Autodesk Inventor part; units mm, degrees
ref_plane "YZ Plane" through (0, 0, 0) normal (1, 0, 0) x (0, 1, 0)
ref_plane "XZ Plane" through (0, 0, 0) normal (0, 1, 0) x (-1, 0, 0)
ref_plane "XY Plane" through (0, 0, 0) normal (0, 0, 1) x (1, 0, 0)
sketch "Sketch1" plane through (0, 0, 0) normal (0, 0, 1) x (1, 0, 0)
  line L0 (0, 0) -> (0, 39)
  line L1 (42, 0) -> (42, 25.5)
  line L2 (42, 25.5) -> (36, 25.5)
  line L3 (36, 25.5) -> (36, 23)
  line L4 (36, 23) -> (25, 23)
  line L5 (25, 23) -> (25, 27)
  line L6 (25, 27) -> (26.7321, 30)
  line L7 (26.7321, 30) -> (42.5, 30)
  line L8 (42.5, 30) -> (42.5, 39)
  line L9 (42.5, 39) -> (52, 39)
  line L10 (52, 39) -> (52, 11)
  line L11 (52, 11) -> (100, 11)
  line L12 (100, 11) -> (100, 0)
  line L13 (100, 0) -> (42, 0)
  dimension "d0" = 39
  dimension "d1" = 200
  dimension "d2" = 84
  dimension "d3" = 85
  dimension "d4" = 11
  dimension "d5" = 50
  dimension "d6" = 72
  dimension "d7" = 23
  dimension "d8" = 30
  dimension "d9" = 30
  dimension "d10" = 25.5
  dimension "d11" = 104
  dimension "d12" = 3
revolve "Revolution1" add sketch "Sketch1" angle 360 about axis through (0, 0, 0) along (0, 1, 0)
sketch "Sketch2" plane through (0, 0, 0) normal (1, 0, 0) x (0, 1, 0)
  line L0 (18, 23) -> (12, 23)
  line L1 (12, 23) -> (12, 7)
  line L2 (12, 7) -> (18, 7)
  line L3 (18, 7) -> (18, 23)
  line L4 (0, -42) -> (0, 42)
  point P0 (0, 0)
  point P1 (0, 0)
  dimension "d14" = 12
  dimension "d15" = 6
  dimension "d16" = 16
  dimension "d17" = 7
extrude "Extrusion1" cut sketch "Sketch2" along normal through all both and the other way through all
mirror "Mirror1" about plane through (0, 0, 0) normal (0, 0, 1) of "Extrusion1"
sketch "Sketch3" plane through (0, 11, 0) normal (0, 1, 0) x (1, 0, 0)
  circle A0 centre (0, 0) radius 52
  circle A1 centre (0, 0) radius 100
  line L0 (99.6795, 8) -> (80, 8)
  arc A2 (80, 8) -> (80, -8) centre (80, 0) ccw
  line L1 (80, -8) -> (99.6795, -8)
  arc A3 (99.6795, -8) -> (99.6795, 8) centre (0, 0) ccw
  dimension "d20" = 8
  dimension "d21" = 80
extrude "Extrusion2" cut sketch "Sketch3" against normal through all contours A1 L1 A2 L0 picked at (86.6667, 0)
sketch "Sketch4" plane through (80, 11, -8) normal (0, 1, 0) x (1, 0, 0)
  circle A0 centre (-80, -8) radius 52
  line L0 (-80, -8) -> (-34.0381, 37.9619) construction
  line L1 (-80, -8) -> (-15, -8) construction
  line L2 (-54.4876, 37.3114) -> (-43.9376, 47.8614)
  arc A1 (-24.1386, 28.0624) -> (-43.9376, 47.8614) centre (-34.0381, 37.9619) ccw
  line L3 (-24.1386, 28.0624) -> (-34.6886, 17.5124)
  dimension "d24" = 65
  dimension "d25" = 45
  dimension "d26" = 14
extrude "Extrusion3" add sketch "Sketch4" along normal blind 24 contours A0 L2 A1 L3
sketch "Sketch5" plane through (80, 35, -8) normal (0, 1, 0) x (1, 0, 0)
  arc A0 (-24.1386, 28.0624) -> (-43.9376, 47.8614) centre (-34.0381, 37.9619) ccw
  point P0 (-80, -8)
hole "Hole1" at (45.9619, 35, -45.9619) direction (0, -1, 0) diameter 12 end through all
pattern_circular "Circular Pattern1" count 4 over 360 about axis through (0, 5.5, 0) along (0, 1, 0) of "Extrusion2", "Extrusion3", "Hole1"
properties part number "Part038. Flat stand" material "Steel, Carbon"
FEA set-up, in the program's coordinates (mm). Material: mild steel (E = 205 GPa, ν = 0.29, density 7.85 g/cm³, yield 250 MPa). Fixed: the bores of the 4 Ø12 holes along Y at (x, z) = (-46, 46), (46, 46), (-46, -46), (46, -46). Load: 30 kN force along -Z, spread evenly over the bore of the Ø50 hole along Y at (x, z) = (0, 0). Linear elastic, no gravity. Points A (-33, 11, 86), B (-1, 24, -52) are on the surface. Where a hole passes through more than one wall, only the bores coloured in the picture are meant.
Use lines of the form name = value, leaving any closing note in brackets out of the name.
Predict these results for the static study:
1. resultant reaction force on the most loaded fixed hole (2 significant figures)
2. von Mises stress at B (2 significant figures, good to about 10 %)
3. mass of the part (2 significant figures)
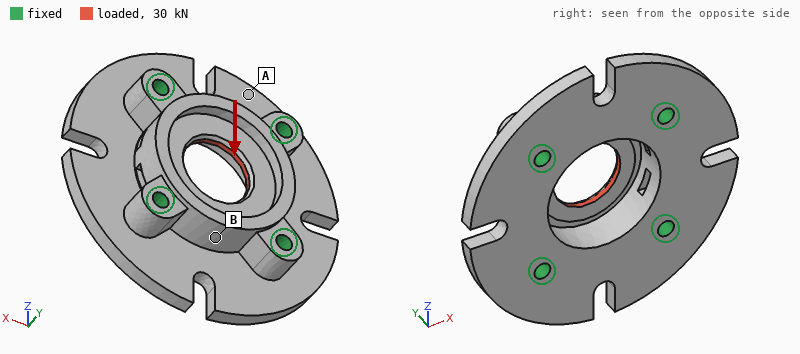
resultant reaction force on the most loaded fixed hole = 7.7 kN
von Mises stress at B = 18 MPa
mass of the part = 3.3 kg
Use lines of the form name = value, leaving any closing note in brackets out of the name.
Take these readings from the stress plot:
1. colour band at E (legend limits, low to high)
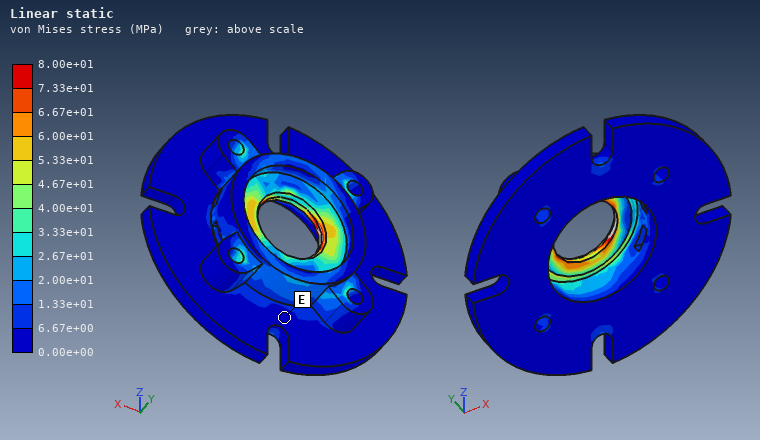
colour band at E = 0.00e+00 to 6.67e+00 MPa
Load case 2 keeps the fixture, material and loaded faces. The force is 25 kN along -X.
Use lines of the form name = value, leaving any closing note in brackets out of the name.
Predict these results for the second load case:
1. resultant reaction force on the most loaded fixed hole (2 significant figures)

resultant reaction force on the most loaded fixed hole = 6.5 kN
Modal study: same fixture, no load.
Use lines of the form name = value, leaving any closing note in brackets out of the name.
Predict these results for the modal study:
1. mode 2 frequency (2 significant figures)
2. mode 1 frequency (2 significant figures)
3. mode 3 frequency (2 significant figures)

mode 2 frequency = 4400 Hz
mode 1 frequency = 4200 Hz
mode 3 frequency = 4500 Hz
